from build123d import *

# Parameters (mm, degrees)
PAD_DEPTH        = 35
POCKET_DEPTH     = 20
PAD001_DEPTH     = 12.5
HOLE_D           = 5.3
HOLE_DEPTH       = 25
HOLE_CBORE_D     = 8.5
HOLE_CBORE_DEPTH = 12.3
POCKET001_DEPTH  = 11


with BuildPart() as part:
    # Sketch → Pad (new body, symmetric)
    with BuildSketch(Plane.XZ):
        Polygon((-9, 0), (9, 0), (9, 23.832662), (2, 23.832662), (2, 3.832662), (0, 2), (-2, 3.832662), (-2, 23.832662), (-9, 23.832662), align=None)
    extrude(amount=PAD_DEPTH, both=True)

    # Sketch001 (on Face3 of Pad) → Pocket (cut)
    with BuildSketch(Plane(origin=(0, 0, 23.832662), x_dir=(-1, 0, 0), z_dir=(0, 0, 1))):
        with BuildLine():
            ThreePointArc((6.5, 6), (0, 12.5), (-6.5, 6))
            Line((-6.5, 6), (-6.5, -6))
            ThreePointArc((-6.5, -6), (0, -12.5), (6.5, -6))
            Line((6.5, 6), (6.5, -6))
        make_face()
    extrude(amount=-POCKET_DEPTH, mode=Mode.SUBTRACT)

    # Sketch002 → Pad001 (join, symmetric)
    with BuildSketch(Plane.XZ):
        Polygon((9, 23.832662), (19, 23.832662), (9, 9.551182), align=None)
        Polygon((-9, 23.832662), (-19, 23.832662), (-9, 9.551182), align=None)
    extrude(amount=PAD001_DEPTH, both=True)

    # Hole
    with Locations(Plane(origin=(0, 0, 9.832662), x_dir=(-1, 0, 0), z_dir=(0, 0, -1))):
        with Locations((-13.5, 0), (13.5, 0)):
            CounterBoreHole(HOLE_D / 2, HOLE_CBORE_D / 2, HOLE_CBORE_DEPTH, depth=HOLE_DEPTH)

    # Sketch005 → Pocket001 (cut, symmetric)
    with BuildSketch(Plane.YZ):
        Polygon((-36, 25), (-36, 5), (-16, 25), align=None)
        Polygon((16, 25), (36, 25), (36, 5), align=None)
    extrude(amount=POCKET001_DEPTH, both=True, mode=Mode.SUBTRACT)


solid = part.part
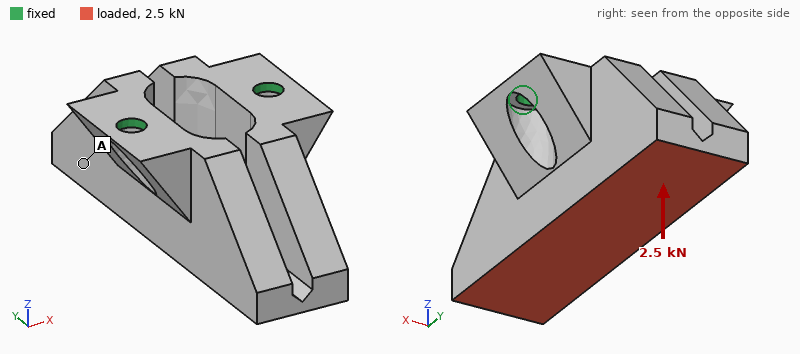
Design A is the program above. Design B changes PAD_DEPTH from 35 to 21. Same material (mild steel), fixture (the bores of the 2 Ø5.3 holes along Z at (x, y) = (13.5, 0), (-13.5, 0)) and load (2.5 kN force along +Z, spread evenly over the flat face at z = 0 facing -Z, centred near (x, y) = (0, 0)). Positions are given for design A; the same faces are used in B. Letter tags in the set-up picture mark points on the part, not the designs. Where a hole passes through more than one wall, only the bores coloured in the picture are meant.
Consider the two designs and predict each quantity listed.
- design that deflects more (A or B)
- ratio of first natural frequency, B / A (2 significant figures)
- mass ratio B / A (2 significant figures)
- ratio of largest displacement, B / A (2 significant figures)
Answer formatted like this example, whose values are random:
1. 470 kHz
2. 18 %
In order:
1. A
2. 1.5
3. 0.71
4. 0.76
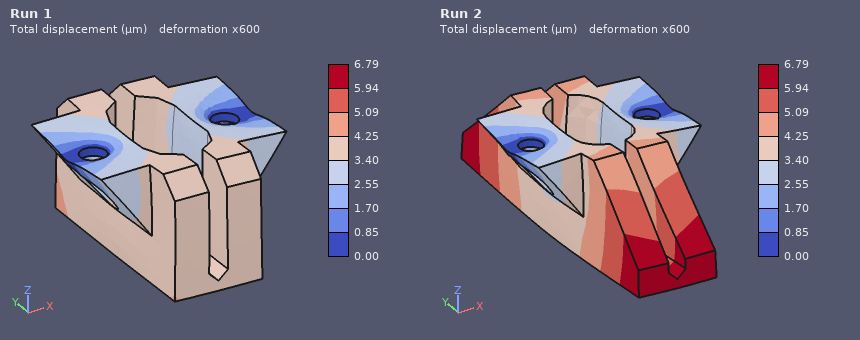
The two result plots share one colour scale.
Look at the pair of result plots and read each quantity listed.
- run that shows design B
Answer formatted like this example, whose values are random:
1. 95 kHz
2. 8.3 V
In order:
1. Run 1
